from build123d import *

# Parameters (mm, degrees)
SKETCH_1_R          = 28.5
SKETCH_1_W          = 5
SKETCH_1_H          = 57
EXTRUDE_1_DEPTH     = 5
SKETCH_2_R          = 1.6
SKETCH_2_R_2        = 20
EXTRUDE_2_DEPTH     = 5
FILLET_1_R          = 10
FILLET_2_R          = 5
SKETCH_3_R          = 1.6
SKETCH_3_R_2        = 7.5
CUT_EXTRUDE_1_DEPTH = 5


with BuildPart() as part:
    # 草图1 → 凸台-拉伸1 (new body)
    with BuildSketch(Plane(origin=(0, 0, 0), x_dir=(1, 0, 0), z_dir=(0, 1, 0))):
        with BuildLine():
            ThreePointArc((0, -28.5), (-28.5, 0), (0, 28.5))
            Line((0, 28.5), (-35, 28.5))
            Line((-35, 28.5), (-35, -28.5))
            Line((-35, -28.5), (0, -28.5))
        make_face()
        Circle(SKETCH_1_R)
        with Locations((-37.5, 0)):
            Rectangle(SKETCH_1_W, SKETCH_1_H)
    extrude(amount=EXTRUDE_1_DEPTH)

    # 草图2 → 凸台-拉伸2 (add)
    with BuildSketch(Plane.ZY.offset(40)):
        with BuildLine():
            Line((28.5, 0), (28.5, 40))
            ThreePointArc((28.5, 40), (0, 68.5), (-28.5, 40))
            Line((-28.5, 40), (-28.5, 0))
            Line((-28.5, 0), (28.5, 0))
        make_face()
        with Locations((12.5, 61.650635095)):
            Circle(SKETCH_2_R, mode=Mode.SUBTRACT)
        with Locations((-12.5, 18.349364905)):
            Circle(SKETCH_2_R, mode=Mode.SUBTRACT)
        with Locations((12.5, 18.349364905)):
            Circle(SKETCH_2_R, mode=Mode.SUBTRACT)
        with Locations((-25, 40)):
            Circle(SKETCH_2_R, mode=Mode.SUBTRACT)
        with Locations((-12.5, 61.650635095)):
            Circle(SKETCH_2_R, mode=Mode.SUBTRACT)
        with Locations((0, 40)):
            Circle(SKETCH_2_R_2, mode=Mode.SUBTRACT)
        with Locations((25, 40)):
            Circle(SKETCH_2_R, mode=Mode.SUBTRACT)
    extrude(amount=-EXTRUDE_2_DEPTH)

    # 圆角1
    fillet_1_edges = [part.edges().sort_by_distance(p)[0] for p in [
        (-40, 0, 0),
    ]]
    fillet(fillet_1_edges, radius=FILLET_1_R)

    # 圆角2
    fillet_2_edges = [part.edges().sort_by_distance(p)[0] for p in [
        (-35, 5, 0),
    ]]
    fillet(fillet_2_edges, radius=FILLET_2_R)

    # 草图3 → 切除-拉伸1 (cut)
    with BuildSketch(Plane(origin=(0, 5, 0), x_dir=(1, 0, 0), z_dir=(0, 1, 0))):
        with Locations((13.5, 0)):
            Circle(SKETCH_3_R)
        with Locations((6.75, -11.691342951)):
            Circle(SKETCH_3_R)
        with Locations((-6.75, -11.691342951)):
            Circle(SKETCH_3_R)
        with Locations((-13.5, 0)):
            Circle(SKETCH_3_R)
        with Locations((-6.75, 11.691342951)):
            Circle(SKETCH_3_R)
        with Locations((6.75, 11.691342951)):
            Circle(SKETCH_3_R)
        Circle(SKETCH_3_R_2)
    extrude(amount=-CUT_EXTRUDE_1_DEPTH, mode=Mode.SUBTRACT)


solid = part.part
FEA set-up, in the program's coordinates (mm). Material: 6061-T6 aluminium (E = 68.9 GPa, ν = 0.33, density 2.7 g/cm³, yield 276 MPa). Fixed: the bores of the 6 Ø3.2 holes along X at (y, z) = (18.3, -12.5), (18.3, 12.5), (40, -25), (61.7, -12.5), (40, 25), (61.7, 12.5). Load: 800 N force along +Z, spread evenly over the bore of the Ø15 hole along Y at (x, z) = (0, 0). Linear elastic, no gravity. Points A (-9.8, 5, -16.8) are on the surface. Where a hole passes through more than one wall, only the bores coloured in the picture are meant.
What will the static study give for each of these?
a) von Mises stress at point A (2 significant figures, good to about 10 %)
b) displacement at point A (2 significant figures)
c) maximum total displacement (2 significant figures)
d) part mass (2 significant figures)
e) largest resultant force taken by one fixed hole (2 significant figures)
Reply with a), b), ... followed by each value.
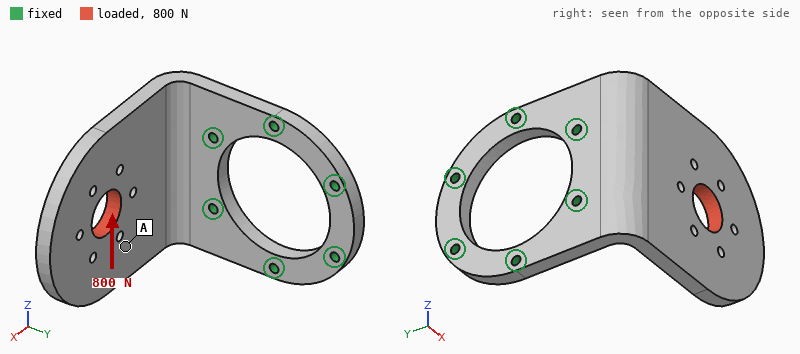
a) 13 MPa
b) 0.10 mm
c) 0.20 mm
d) 69 g
e) 1.1 kN
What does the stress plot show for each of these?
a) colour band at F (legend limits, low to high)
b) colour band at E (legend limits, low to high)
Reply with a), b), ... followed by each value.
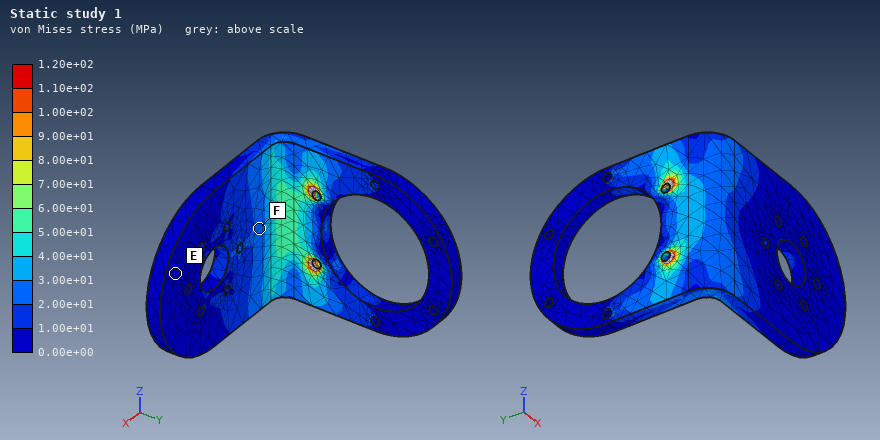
a) 2.00e+01 to 3.00e+01 MPa
b) 0.00e+00 to 1.00e+01 MPa
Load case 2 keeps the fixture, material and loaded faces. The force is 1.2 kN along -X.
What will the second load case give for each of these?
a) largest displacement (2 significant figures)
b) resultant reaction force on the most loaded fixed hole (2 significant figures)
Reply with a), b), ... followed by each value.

a) 0.33 mm
b) 710 N
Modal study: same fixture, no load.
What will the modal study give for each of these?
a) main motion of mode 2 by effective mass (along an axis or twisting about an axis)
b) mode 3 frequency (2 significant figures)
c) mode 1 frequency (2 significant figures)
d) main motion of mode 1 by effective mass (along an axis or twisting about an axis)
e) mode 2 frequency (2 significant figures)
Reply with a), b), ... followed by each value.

a) along Z
b) 3100 Hz
c) 820 Hz
d) along Y
e) 1900 Hz
